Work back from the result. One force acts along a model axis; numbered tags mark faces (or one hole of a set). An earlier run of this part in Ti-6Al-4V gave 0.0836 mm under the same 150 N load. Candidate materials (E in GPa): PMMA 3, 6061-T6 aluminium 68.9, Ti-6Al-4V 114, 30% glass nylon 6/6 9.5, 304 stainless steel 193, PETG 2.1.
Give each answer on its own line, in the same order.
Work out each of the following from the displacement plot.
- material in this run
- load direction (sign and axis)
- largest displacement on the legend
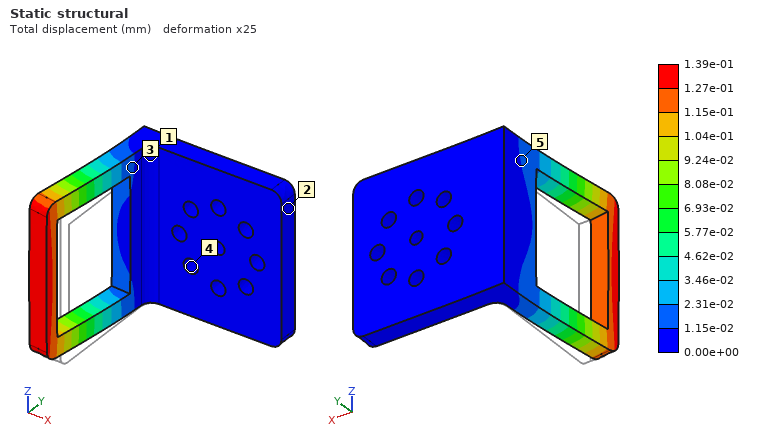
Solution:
6061-T6 aluminium
-X
1.39e-01 mm
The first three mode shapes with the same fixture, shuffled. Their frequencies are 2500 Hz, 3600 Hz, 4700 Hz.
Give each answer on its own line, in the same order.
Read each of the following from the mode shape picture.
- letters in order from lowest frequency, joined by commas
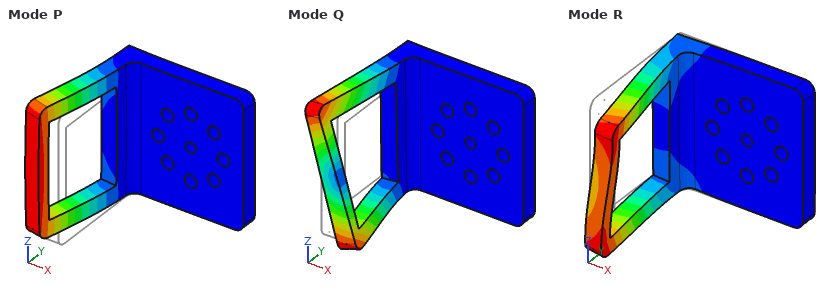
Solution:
P, R, Q
